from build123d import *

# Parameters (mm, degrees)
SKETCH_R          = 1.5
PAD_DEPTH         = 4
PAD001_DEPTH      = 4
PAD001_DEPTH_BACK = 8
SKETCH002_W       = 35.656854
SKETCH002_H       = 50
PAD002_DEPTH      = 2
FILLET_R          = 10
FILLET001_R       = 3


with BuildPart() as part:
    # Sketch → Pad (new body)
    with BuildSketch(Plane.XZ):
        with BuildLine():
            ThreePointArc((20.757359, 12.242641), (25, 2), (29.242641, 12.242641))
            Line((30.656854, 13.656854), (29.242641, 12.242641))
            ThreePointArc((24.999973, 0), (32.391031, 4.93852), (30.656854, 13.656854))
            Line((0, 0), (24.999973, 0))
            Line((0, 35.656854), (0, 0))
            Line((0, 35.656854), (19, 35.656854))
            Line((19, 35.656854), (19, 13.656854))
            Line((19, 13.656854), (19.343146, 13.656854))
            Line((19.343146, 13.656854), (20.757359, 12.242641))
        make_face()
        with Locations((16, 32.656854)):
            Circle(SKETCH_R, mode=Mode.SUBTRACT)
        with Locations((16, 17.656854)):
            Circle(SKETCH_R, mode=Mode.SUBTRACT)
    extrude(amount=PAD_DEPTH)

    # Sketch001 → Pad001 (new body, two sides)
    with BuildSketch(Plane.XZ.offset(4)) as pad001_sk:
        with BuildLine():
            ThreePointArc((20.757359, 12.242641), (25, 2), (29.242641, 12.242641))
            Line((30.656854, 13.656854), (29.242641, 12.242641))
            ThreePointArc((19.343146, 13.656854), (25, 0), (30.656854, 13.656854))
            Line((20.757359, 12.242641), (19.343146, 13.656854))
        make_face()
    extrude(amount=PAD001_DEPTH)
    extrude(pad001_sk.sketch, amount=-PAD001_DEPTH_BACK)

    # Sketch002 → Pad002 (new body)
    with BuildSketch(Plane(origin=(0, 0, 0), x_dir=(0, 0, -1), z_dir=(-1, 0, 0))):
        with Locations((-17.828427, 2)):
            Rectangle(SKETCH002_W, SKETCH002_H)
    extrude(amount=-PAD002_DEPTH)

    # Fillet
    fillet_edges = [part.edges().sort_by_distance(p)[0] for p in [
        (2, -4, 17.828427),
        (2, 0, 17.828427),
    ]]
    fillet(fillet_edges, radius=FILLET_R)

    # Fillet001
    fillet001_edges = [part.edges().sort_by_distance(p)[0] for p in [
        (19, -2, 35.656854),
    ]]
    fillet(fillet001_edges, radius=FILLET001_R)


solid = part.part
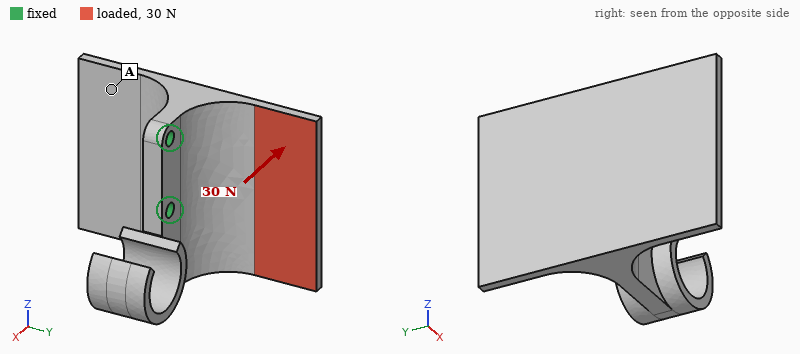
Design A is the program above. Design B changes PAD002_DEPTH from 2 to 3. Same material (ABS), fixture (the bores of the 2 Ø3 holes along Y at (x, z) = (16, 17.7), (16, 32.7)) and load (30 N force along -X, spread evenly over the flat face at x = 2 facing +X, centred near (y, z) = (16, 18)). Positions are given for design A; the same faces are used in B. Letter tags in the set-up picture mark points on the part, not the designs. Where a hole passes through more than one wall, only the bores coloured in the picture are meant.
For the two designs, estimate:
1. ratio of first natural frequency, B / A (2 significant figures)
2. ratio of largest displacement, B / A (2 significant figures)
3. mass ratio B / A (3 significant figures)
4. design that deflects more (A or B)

0.93
0.63
1.20
A
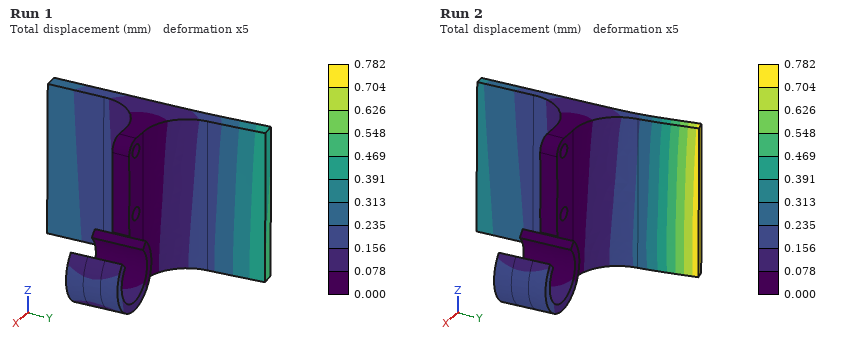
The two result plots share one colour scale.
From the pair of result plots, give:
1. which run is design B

Run 1
